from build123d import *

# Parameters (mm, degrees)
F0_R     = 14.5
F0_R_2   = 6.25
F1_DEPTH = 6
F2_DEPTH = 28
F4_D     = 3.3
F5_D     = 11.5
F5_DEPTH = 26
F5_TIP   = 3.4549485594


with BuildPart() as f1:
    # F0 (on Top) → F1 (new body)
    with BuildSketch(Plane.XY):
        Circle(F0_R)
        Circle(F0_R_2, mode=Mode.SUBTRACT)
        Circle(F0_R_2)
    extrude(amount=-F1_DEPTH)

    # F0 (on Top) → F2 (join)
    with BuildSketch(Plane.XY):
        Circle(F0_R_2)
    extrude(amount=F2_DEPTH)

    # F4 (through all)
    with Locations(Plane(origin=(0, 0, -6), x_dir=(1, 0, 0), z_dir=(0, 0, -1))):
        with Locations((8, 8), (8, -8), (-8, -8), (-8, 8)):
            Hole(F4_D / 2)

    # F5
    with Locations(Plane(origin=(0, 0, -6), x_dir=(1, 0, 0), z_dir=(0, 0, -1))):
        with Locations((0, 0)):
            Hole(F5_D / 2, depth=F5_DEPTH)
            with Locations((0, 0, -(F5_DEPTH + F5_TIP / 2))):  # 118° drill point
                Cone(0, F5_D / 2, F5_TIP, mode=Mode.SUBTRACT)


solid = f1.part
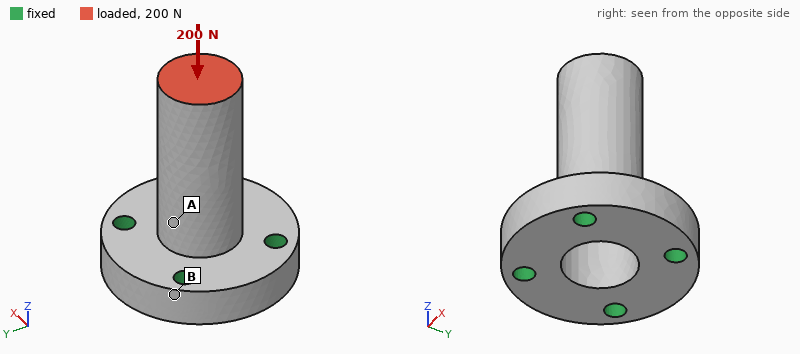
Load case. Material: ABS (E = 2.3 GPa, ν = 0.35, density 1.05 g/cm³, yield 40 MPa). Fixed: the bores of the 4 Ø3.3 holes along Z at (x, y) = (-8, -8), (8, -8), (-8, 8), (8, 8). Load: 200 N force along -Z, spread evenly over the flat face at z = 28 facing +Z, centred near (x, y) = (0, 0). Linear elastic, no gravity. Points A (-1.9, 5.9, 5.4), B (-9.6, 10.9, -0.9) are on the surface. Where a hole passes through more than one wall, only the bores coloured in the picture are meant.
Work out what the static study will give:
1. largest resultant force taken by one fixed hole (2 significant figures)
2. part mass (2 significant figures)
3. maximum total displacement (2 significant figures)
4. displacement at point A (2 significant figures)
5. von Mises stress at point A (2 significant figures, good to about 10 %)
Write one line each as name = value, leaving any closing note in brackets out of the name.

largest resultant force taken by one fixed hole = 51 N
part mass = 4.6 g
maximum total displacement = 0.12 mm
displacement at point A = 0.038 mm
von Mises stress at point A = 11 MPa
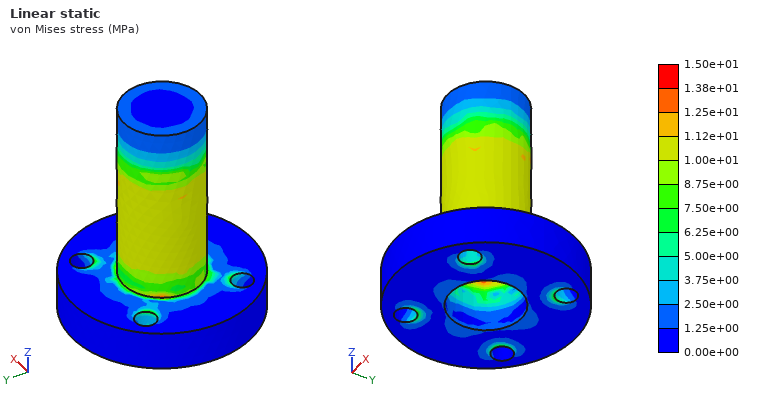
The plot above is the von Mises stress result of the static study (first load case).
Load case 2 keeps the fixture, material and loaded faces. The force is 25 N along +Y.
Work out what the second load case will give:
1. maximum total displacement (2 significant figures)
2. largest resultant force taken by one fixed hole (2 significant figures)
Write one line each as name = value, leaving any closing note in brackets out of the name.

maximum total displacement = 0.36 mm
largest resultant force taken by one fixed hole = 31 N
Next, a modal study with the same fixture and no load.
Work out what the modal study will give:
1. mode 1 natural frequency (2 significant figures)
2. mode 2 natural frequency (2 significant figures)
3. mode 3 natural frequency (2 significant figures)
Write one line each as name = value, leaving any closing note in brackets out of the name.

mode 1 natural frequency = 1600 Hz
mode 2 natural frequency = 1600 Hz
mode 3 natural frequency = 5300 Hz
